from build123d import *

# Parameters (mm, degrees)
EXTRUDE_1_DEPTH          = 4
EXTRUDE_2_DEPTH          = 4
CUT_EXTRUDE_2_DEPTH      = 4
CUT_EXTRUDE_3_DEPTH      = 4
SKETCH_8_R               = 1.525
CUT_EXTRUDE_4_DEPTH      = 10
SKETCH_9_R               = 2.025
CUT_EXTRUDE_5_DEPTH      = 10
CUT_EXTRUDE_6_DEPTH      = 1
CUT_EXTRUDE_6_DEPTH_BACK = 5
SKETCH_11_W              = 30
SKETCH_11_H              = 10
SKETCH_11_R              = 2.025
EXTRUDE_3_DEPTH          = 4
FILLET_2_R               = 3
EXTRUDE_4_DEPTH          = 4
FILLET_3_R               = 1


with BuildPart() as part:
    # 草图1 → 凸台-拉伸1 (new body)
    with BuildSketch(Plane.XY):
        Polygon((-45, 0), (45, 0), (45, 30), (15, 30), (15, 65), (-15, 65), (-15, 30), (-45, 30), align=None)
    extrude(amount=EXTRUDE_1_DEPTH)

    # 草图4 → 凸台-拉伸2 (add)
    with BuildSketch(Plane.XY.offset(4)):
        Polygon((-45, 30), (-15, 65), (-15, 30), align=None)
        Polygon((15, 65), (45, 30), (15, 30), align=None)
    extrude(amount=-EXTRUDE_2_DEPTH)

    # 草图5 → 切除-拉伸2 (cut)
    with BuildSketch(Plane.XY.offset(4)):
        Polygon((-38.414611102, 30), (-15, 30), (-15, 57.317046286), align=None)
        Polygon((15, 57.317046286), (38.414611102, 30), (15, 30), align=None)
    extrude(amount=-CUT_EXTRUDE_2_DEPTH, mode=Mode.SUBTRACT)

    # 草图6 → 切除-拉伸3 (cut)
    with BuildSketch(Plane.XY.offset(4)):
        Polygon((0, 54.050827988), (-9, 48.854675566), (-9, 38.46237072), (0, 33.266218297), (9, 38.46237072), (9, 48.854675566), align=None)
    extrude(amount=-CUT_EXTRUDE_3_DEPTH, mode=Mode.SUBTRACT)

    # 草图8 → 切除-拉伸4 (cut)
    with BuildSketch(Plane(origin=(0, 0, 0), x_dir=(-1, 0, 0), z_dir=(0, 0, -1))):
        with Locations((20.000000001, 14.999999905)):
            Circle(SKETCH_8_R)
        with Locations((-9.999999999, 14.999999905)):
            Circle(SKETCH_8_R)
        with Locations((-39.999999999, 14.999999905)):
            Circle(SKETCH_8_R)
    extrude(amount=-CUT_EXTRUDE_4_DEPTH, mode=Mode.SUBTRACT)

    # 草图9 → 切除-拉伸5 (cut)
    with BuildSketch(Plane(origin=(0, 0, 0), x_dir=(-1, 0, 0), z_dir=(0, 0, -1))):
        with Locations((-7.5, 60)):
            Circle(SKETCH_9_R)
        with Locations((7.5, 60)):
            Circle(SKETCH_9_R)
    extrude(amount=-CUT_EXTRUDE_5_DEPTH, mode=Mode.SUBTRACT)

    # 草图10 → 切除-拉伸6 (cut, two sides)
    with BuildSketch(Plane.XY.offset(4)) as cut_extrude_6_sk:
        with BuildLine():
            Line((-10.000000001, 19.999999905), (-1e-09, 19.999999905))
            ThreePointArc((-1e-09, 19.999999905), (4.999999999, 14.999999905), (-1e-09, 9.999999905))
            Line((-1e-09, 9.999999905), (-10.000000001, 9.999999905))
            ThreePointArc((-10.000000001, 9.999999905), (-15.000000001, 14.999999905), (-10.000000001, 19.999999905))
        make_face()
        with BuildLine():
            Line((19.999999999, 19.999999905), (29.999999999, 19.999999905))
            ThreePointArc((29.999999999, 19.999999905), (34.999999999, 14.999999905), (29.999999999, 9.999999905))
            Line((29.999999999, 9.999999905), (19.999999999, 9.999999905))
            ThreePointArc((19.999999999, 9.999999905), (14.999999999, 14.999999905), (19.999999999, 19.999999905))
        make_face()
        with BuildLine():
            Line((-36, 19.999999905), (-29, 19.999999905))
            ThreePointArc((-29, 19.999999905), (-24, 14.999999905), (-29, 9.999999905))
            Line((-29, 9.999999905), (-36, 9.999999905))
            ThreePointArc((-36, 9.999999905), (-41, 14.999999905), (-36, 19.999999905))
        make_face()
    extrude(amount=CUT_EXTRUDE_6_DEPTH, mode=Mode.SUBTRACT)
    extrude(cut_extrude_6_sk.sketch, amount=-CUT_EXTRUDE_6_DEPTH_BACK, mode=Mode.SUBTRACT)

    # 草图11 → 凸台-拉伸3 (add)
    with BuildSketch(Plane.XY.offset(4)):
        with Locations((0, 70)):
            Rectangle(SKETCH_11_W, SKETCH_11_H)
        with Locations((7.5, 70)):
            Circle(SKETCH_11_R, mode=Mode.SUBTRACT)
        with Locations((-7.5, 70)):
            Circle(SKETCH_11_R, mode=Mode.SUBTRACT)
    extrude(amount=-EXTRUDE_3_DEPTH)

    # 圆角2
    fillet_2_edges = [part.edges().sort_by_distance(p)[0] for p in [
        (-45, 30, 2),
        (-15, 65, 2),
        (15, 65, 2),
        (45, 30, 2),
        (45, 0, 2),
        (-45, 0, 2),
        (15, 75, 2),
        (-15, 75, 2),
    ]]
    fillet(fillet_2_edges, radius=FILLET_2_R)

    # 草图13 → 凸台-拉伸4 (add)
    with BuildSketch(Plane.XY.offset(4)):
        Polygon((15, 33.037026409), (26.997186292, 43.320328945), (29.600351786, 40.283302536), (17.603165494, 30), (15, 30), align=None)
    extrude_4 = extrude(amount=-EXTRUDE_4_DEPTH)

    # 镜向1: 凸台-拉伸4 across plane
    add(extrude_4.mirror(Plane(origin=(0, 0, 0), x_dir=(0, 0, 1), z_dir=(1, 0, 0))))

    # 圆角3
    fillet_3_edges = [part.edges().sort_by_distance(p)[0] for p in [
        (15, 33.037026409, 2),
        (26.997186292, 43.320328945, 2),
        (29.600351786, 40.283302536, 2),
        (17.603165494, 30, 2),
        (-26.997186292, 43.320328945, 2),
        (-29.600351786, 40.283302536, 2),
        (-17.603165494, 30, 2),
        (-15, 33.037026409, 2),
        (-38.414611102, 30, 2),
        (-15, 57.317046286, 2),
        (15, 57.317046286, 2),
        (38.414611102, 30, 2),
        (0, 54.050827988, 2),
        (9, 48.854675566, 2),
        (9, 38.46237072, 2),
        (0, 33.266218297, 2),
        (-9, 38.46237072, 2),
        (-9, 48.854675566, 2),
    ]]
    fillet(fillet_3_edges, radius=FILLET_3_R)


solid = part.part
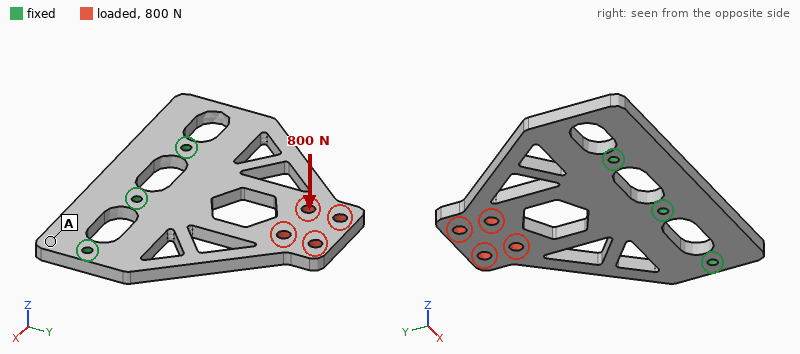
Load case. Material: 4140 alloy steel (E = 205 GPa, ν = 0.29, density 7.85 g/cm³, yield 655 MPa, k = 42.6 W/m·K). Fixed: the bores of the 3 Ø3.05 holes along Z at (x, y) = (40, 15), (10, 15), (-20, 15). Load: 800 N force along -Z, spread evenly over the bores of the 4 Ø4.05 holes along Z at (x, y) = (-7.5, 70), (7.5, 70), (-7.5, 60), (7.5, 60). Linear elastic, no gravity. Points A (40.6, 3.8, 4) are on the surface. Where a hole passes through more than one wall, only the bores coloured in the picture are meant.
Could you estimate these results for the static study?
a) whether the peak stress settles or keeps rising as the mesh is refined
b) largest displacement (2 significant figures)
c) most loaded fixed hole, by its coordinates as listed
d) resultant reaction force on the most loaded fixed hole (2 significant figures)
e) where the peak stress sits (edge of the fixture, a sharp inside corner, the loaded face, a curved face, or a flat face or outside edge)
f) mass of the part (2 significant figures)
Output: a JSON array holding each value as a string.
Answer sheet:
["keeps rising", "1.2 mm", "(10, 15)", "460 N", "edge of the fixture", "120 g"]
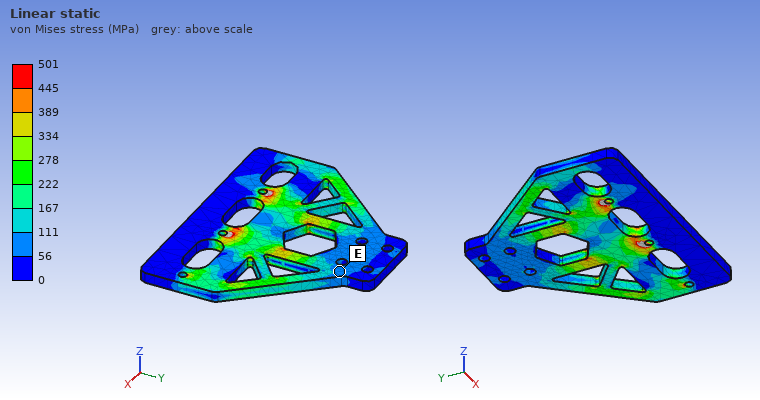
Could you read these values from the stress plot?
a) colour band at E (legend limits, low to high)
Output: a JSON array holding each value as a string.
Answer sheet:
["56 to 111 MPa"]
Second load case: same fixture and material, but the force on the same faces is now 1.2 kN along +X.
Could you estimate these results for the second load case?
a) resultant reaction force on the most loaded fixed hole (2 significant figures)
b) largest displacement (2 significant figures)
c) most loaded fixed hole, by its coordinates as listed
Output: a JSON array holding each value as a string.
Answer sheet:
["1.1 kN", "17 µm", "(-20, 15)"]
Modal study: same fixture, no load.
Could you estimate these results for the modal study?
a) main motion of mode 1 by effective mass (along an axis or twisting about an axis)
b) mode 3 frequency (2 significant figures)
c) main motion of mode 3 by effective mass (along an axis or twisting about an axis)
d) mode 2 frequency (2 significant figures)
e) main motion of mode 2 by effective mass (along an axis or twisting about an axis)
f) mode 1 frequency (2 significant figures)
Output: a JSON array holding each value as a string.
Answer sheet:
["along Z", "4000 Hz", "along Z", "3000 Hz", "twisting about Y", "980 Hz"]
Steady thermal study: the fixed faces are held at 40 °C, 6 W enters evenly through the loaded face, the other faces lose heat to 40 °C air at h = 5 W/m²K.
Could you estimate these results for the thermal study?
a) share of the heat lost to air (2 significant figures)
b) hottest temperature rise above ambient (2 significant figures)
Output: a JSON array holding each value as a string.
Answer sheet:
["15 %", "58 K"]
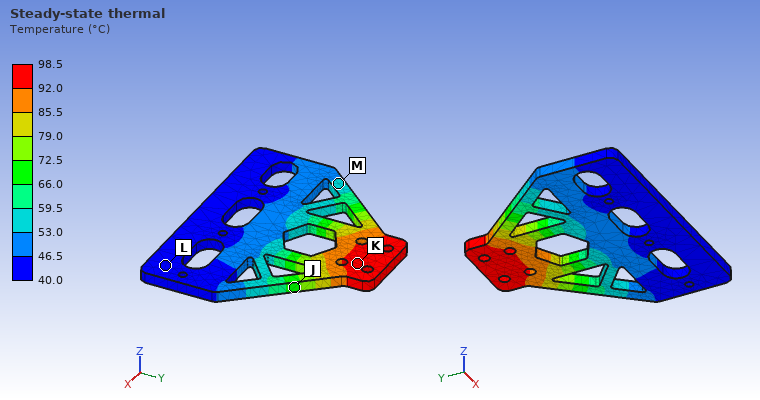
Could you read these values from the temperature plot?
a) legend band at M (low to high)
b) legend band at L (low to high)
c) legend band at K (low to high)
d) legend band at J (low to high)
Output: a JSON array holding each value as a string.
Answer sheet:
["53.0 to 59.5 °C", "40.0 to 46.5 °C", "92.0 to 98.5 °C", "66.0 to 72.5 °C"]
